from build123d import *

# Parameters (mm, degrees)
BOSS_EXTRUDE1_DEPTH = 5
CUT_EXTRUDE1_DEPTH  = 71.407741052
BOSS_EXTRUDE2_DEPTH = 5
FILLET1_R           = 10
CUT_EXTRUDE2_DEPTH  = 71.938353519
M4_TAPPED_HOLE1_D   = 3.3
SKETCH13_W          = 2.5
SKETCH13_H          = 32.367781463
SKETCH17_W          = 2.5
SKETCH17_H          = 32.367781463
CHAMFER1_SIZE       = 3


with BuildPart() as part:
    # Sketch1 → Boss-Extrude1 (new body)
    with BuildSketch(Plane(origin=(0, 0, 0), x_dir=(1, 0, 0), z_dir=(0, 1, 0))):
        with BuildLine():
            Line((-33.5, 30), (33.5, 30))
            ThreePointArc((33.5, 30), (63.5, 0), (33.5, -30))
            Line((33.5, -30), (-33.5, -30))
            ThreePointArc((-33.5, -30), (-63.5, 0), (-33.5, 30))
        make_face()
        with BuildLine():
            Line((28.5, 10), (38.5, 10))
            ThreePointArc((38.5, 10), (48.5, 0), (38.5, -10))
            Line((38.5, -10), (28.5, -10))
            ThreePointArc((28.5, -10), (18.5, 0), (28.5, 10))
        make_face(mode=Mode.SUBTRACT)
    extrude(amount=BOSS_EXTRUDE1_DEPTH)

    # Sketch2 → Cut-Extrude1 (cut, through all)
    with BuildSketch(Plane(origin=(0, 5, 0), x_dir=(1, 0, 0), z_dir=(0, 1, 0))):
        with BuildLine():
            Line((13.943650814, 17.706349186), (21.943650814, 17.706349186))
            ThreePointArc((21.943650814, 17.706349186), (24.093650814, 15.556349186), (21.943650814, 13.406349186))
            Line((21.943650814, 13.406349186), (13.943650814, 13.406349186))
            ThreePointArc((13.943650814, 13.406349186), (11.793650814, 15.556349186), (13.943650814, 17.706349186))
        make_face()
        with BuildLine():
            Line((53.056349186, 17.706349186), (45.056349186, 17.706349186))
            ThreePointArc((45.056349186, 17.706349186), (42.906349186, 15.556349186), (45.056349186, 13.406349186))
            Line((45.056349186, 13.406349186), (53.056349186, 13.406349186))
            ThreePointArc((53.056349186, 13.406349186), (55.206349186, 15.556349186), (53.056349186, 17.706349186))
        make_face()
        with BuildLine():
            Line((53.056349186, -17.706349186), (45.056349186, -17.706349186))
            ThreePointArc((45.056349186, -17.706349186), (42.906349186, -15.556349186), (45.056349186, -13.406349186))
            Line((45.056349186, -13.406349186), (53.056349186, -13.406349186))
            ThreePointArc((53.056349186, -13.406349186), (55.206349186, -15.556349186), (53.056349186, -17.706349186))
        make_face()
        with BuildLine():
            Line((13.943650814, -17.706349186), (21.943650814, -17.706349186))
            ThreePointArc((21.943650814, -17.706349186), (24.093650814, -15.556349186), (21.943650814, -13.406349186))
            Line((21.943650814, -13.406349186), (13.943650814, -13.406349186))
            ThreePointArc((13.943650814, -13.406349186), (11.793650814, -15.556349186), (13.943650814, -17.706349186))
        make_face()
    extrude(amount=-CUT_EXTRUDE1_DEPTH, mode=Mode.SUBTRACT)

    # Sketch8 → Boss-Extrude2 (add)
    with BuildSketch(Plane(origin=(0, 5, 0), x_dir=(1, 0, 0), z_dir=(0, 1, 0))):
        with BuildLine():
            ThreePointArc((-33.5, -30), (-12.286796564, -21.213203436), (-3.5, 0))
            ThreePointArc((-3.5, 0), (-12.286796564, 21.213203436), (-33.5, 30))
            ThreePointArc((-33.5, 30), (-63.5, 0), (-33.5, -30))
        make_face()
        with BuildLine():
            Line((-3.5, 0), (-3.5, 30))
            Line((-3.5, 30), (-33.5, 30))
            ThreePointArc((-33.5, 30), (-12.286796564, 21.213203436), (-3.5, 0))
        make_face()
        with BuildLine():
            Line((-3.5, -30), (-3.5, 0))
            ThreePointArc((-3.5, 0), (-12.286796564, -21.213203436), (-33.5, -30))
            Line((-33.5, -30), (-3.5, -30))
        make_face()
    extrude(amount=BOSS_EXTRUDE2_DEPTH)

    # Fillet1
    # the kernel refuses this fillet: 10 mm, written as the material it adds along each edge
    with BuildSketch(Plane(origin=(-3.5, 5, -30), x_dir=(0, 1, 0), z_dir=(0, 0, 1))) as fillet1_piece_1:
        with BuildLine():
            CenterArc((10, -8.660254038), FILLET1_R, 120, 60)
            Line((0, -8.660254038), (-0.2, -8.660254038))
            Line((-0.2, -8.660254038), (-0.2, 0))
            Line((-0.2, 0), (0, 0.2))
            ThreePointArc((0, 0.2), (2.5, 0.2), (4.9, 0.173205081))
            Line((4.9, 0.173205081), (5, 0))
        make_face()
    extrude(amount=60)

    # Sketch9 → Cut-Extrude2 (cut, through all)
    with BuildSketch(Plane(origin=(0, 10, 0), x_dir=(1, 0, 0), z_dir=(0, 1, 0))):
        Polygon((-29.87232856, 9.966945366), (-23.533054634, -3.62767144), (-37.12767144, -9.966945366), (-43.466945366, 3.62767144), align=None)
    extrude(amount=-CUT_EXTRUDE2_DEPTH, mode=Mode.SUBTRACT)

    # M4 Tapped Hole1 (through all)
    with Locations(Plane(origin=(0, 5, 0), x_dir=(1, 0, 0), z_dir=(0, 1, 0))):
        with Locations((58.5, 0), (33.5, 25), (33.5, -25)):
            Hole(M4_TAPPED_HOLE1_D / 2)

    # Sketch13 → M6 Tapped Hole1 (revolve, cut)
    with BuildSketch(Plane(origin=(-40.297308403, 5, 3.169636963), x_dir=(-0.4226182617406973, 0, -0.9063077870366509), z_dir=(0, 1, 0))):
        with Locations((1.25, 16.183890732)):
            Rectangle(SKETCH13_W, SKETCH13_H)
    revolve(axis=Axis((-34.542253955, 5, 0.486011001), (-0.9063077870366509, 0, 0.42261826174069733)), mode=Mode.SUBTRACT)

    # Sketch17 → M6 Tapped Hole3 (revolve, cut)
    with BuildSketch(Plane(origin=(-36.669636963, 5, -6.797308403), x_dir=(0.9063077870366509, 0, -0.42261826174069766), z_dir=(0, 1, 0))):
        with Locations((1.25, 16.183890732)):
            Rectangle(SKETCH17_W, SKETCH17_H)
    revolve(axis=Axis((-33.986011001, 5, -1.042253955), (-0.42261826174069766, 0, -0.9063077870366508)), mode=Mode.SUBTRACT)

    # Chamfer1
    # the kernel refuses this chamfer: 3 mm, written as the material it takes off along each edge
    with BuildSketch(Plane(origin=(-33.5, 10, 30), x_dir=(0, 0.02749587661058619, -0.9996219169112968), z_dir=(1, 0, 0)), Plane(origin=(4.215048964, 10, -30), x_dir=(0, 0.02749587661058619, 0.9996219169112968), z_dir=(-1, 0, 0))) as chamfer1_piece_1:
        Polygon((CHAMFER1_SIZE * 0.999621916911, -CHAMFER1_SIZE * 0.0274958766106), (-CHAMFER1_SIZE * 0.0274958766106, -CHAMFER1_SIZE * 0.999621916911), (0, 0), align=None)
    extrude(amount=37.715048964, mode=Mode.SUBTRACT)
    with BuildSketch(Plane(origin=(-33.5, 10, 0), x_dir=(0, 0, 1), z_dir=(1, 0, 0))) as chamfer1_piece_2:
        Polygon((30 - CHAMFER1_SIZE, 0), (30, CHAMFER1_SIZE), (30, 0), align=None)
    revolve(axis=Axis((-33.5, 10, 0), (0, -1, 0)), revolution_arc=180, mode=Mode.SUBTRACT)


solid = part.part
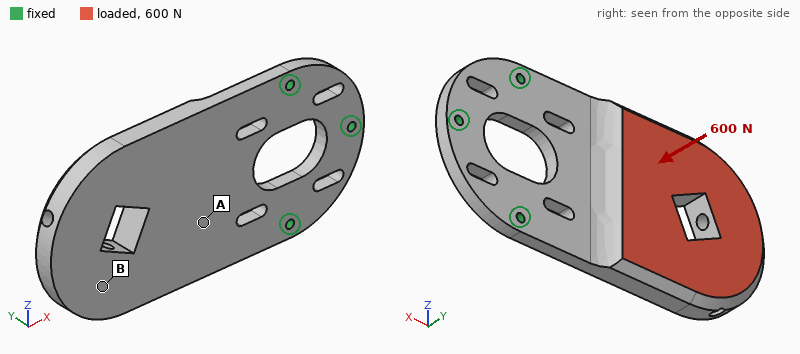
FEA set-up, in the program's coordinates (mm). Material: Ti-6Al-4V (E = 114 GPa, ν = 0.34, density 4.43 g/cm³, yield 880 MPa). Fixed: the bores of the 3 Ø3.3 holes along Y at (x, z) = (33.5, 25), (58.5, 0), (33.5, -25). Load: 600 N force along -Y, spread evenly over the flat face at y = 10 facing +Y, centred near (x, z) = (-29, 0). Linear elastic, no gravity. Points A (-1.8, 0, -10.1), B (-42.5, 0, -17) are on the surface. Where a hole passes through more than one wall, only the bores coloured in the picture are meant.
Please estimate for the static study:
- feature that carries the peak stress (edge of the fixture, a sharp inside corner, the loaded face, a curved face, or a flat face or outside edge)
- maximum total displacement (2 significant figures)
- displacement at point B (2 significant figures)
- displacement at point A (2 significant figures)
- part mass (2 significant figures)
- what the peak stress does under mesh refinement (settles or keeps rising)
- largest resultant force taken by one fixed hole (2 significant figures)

edge of the fixture
1.6 mm
1.2 mm
0.44 mm
190 g
keeps rising
500 N
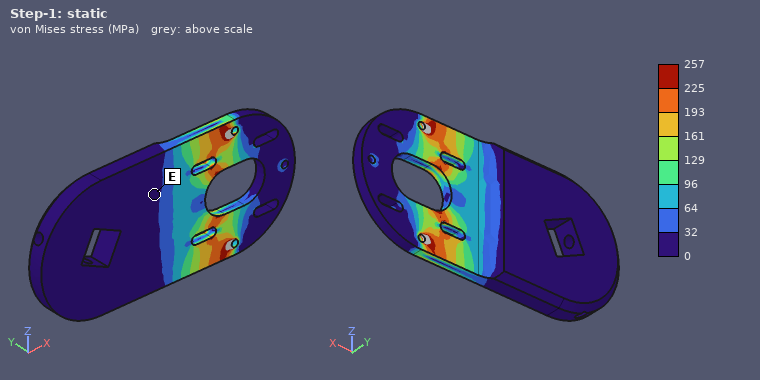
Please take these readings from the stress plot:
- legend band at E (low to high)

0 to 32 MPa
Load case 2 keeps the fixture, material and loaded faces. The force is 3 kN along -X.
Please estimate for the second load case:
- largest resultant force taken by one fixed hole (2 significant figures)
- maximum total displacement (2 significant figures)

1.4 kN
1.2 mm
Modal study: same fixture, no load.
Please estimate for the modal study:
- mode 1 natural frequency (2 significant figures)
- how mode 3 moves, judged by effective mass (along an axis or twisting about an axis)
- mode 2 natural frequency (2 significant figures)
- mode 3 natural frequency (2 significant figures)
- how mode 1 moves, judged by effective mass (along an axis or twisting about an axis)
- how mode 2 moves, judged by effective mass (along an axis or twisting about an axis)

330 Hz
along Z
1800 Hz
3300 Hz
along Y
twisting about X
